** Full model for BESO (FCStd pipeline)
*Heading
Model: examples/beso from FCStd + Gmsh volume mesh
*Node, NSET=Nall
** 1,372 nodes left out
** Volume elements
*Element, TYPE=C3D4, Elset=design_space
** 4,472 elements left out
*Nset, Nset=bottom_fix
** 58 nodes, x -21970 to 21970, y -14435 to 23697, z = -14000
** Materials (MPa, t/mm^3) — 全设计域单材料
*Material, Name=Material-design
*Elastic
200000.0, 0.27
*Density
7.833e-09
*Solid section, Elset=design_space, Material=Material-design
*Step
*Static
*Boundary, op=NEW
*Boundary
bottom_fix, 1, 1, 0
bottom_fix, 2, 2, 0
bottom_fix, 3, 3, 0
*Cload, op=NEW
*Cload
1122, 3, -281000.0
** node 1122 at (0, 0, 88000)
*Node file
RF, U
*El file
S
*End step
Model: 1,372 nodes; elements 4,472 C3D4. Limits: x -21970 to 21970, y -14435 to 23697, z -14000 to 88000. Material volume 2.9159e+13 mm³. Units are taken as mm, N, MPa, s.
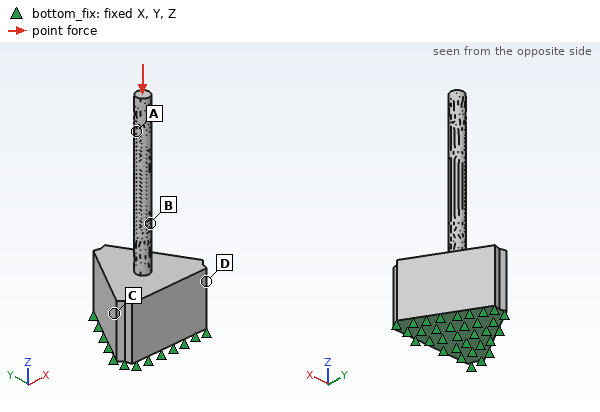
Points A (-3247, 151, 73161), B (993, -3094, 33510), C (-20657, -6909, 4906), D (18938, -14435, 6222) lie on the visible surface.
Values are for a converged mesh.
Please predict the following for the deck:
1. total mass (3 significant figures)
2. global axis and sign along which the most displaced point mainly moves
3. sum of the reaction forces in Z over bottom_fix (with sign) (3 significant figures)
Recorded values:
2.28e+08 kg
-Z
2.81e+05 N
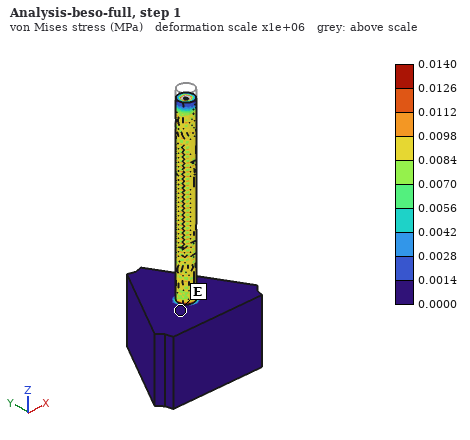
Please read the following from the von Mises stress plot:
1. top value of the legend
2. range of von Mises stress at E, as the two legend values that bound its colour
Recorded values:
0.0140 MPa
0.0000 to 0.0014 MPa
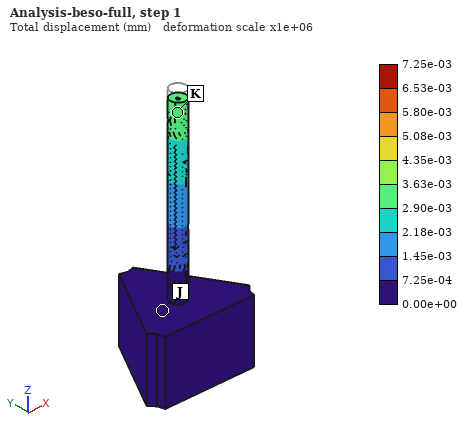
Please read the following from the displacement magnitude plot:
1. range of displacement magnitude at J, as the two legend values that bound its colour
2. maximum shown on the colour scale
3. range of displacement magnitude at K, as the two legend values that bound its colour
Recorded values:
0.00e+00 to 7.25e-04 mm
7.25e-03 mm
2.90e-03 to 3.63e-03 mm
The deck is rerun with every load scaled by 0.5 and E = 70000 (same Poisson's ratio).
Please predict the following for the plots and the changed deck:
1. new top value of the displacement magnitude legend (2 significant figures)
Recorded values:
0.010 mm
